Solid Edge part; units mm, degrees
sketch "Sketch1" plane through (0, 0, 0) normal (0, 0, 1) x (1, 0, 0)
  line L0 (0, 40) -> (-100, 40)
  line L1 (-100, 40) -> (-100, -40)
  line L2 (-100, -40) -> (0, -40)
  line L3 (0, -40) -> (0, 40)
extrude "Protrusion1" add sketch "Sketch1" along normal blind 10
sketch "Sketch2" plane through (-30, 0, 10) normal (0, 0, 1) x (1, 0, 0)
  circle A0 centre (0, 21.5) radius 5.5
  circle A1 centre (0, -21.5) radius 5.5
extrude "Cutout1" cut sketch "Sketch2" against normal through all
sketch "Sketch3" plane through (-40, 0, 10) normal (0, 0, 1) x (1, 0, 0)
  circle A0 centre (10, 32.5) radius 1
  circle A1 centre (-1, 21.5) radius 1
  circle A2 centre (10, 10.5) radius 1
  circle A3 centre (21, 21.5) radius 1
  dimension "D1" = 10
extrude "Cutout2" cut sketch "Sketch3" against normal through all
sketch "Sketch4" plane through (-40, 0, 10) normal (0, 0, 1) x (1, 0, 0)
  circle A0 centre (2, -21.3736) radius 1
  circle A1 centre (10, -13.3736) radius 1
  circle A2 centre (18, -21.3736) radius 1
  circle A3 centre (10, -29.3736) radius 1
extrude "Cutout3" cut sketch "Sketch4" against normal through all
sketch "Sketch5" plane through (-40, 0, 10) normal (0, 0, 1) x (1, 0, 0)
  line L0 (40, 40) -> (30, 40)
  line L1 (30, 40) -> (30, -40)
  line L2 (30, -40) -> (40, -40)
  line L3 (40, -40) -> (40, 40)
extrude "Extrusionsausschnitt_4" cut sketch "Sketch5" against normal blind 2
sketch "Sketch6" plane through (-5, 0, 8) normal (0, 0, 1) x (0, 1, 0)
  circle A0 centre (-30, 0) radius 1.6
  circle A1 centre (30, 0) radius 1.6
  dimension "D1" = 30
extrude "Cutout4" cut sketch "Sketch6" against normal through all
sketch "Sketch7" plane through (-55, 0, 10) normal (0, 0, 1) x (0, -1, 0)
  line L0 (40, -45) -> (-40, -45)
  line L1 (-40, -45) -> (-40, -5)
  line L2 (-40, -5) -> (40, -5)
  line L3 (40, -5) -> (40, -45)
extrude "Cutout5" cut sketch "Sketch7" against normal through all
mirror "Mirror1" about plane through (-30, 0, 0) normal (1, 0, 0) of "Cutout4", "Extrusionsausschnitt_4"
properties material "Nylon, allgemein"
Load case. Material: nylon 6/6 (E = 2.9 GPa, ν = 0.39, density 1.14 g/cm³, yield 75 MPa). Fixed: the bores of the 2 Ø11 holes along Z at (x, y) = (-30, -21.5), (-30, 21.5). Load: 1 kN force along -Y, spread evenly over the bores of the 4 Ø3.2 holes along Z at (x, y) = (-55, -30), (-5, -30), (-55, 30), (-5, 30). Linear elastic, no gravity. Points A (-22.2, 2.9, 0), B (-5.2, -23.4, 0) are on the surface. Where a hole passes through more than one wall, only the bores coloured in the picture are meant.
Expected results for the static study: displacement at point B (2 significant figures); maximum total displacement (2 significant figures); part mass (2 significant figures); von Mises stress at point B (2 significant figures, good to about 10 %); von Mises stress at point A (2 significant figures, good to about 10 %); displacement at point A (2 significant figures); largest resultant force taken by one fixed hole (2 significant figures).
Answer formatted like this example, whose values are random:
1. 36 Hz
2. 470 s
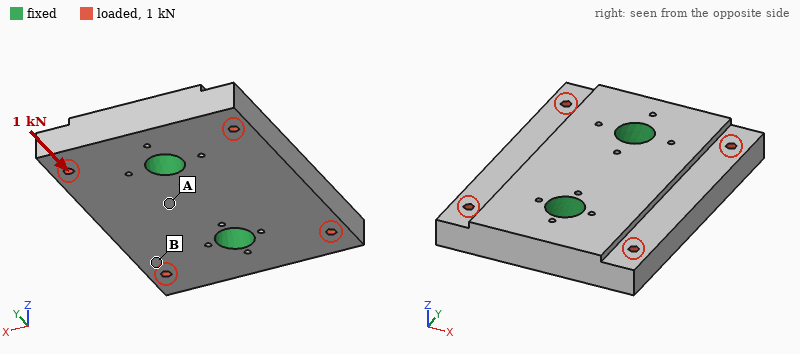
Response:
1. 22 µm
2. 35 µm
3. 48 g
4. 2.3 MPa
5. 1.0 MPa
6. 6.1 µm
7. 500 N
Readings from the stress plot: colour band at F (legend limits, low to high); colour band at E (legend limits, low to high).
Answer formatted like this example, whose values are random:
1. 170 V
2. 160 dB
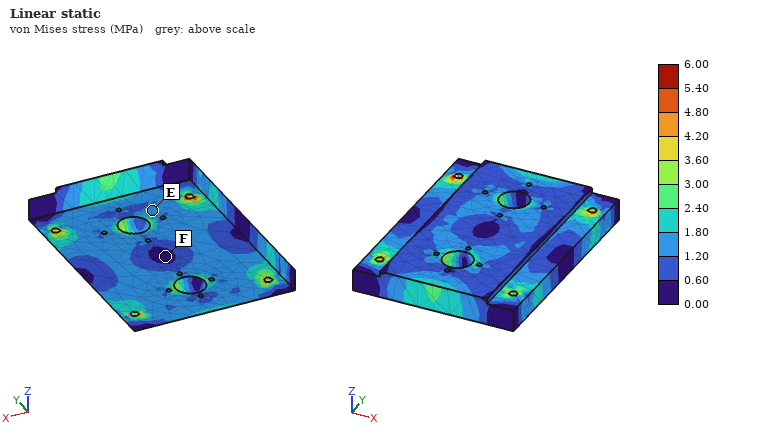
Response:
1. 0.00 to 0.60 MPa
2. 1.20 to 1.80 MPa
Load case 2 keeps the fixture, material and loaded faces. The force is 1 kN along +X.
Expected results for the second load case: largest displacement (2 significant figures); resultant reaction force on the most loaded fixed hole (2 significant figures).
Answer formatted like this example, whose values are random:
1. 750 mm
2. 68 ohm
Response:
1. 28 µm
2. 500 N
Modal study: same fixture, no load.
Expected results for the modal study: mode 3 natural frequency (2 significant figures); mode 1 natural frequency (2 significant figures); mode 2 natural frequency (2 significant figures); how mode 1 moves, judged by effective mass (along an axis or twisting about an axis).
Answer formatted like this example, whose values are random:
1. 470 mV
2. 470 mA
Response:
1. 3500 Hz
2. 2900 Hz
3. 3400 Hz
4. twisting about Y
